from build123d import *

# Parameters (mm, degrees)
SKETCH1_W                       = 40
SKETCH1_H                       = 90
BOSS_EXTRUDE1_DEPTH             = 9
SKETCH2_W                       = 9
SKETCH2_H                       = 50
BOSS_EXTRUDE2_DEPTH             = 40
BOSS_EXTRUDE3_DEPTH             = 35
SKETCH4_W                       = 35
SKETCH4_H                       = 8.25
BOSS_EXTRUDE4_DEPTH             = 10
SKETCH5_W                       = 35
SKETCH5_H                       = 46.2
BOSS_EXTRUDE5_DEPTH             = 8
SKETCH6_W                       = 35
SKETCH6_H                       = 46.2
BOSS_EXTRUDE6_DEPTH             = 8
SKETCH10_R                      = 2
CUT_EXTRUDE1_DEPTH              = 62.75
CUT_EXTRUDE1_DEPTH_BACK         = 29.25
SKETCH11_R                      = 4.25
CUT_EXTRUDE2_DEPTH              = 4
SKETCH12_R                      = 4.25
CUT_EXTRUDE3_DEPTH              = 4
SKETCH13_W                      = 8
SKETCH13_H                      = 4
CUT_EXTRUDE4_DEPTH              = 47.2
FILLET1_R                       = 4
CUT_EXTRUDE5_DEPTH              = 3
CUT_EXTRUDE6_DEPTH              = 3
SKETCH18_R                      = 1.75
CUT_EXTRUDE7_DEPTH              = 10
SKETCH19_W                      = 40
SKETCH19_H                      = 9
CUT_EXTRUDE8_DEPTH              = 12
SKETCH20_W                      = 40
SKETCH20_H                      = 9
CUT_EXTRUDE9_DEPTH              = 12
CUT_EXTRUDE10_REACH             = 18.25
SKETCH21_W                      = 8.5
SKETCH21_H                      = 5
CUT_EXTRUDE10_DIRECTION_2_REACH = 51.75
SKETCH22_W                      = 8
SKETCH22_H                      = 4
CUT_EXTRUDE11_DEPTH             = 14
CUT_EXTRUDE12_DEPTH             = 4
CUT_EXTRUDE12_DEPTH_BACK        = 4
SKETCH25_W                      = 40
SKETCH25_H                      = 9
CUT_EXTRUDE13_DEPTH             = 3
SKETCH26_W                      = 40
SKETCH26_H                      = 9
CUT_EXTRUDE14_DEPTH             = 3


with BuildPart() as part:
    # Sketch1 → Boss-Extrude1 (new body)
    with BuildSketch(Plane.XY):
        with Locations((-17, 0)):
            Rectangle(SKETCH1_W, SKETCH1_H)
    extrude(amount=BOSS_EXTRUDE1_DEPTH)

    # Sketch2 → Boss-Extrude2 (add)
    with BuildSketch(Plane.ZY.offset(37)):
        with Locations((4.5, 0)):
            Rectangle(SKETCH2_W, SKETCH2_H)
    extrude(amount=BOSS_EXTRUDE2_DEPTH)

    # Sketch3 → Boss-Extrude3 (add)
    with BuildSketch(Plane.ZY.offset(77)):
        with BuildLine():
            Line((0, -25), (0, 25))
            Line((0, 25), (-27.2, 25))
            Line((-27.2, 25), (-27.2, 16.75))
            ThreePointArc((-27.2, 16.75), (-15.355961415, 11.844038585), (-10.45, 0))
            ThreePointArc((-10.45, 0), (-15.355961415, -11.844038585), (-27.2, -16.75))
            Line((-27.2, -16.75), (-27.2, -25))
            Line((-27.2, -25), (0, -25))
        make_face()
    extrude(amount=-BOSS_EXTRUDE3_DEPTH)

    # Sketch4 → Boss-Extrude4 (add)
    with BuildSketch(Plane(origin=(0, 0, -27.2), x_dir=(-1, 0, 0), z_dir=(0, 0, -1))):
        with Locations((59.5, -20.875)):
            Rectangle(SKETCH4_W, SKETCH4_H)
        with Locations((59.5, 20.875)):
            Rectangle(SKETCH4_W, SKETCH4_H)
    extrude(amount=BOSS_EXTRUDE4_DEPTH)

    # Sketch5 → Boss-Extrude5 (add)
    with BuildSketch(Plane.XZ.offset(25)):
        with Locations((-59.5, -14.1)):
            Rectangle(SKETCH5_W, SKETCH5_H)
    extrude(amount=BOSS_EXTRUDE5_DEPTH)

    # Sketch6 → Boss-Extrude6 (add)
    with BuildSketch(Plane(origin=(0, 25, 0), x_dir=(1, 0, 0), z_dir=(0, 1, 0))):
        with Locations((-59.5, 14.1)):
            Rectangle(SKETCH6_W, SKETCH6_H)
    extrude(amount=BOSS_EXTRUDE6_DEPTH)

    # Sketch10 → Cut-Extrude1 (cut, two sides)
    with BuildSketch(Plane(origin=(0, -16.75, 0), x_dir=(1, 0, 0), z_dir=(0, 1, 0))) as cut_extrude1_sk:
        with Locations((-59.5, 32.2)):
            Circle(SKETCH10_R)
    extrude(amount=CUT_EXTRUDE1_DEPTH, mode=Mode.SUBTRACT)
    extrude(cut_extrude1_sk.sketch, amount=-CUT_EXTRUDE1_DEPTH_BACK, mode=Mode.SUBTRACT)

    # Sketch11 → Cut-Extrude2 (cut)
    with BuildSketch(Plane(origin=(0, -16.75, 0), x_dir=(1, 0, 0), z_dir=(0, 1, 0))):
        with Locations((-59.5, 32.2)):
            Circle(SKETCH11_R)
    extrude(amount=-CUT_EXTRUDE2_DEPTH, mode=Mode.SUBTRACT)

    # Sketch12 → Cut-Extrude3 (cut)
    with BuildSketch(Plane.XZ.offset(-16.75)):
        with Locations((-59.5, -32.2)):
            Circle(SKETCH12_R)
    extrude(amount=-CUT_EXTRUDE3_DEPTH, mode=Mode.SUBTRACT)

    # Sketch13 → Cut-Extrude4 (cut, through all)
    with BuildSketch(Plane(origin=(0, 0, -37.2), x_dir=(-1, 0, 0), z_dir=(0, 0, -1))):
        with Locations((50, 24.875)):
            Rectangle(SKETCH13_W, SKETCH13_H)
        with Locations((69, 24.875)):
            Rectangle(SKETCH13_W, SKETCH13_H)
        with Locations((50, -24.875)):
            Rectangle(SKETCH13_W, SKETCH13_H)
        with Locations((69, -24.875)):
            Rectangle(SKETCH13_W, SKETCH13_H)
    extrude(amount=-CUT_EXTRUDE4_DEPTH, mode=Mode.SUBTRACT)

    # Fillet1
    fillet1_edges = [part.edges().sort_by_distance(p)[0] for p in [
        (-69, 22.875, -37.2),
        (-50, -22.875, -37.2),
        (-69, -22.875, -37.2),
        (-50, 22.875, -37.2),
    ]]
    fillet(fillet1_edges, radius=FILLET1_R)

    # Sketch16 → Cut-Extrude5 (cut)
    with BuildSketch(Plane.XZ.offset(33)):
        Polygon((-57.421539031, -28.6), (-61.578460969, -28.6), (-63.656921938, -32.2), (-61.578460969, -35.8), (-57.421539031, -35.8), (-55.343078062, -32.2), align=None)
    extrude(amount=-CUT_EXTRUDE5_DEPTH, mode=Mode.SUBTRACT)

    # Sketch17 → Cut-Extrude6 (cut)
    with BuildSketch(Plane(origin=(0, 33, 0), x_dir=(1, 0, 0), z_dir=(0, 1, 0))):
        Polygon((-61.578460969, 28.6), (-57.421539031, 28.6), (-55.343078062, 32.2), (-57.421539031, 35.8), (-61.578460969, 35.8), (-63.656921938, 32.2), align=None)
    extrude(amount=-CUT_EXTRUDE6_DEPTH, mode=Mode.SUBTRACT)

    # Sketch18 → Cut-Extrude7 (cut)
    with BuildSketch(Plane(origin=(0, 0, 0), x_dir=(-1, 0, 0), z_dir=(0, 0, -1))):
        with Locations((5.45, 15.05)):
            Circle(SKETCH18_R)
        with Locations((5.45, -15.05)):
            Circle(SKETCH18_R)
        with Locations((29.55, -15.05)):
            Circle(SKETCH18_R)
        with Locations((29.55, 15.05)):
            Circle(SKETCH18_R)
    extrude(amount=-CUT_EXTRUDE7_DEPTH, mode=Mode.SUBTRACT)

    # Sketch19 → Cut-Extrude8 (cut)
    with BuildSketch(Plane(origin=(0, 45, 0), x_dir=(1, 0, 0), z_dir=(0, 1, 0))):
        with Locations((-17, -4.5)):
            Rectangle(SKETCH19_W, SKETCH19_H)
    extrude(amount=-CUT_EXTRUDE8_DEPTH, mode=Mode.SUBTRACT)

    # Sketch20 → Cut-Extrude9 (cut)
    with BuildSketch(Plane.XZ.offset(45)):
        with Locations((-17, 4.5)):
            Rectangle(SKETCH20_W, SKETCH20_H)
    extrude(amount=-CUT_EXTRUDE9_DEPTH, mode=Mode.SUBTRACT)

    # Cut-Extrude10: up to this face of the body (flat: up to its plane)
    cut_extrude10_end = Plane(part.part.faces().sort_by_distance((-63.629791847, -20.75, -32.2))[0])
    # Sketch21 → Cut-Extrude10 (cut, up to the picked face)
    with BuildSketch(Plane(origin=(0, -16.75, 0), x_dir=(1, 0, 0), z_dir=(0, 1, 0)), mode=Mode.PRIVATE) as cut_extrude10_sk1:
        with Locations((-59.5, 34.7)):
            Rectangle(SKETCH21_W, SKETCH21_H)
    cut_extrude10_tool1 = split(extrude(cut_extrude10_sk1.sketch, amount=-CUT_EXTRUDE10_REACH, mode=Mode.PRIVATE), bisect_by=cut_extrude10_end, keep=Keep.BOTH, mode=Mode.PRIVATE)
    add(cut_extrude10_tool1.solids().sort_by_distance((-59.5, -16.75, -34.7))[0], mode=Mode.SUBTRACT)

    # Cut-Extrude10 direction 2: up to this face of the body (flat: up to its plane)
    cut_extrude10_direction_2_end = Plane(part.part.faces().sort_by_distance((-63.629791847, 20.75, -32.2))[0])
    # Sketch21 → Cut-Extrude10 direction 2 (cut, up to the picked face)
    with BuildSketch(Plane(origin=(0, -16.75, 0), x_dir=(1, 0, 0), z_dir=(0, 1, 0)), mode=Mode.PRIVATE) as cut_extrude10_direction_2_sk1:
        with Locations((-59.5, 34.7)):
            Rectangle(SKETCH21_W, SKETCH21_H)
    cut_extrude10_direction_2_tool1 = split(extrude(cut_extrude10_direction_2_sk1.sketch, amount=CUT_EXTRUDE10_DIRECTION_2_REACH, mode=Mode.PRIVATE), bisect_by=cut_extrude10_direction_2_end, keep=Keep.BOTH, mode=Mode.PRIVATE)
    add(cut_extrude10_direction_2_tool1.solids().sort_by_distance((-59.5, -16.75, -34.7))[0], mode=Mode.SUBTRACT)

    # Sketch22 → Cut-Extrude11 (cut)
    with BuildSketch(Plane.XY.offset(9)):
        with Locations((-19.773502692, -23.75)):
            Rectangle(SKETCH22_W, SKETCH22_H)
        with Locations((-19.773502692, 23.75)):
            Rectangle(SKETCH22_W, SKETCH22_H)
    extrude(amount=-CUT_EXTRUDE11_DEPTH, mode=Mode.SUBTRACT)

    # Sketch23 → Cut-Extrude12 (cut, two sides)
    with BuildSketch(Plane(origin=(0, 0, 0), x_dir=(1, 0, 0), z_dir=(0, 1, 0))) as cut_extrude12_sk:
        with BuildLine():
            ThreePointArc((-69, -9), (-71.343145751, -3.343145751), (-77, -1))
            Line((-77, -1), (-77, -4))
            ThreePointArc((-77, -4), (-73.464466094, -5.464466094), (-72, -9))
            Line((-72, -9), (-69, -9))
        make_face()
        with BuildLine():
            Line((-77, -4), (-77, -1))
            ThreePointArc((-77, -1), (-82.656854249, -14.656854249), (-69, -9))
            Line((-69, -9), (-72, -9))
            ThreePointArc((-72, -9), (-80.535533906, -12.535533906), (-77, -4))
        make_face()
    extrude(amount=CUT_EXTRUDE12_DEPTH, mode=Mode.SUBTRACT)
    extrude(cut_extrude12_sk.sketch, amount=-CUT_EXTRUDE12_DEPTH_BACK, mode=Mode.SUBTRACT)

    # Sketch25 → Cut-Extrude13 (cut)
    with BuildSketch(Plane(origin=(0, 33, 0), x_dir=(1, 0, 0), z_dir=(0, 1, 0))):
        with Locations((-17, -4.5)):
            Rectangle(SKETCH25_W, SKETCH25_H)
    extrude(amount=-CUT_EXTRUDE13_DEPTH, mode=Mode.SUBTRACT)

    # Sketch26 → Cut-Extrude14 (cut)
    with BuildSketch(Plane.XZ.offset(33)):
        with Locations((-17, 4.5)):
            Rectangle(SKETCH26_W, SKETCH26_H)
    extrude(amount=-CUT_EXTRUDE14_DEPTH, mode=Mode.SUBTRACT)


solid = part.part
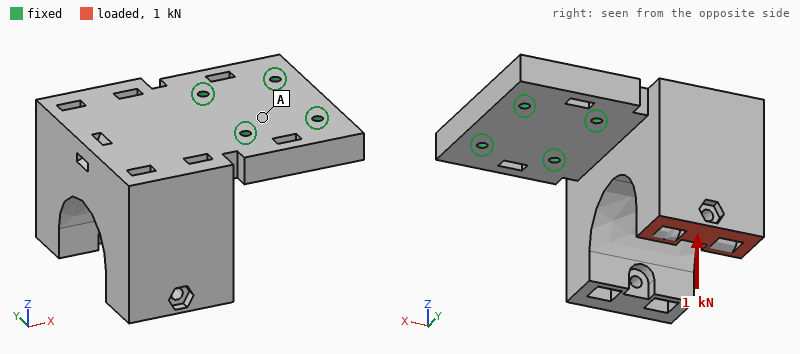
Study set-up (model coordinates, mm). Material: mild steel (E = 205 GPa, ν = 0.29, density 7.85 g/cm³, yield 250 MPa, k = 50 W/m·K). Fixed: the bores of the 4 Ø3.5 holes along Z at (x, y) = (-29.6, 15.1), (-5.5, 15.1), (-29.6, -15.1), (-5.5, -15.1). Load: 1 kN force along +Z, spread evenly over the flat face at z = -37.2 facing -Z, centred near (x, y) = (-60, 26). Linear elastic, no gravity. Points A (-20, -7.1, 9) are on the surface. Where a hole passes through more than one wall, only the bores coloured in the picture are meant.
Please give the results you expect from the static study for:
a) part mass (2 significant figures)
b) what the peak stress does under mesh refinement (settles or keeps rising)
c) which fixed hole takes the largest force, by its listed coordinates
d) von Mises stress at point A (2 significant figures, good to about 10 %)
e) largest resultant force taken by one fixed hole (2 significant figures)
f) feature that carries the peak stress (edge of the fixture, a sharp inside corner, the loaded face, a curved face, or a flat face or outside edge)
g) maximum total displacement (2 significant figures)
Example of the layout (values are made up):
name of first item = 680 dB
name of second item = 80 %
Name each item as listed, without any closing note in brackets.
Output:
part mass = 750 g
what the peak stress does under mesh refinement = keeps rising
which fixed hole takes the largest force, by its listed coordinates = (-29.6, 15.1)
von Mises stress at point A = 7.3 MPa
largest resultant force taken by one fixed hole = 1.5 kN
feature that carries the peak stress = edge of the fixture
maximum total displacement = 45 µm
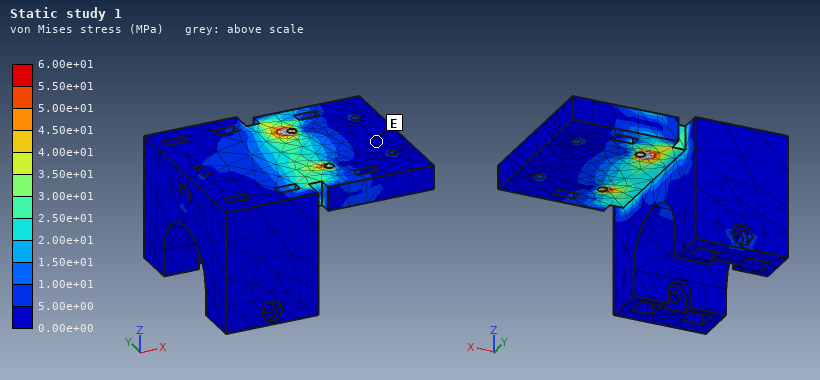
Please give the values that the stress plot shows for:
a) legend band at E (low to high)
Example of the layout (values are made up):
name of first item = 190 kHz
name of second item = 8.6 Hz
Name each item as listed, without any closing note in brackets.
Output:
legend band at E = 0.00e+00 to 5.00e+00 MPa
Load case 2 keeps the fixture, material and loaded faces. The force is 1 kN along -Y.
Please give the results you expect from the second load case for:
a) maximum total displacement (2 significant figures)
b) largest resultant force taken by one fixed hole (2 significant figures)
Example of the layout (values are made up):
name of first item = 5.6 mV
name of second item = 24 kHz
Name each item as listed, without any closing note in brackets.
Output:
maximum total displacement = 21 µm
largest resultant force taken by one fixed hole = 1.5 kN
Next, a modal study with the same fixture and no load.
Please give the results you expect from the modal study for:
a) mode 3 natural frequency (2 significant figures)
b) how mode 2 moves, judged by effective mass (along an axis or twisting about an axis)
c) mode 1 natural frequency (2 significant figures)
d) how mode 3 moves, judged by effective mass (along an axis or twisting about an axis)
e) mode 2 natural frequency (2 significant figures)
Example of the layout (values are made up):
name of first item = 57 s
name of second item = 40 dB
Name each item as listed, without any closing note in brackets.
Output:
mode 3 natural frequency = 4900 Hz
how mode 2 moves, judged by effective mass = along Y
mode 1 natural frequency = 1300 Hz
how mode 3 moves, judged by effective mass = along Y
mode 2 natural frequency = 2900 Hz
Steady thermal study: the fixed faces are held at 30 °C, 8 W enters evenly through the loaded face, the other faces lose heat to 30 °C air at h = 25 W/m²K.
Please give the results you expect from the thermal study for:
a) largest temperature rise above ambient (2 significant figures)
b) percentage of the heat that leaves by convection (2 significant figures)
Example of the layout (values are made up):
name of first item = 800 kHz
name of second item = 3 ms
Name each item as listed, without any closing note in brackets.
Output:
largest temperature rise above ambient = 18 K
percentage of the heat that leaves by convection = 37 %
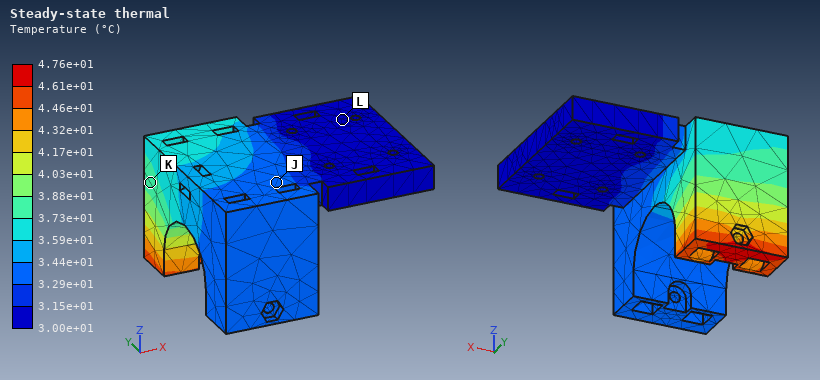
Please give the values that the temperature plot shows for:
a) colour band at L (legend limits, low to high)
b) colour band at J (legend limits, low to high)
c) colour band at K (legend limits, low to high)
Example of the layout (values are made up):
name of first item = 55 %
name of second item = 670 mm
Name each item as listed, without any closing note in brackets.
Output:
colour band at L = 3.00e+01 to 3.15e+01 °C
colour band at J = 3.29e+01 to 3.44e+01 °C
colour band at K = 3.73e+01 to 3.88e+01 °C
